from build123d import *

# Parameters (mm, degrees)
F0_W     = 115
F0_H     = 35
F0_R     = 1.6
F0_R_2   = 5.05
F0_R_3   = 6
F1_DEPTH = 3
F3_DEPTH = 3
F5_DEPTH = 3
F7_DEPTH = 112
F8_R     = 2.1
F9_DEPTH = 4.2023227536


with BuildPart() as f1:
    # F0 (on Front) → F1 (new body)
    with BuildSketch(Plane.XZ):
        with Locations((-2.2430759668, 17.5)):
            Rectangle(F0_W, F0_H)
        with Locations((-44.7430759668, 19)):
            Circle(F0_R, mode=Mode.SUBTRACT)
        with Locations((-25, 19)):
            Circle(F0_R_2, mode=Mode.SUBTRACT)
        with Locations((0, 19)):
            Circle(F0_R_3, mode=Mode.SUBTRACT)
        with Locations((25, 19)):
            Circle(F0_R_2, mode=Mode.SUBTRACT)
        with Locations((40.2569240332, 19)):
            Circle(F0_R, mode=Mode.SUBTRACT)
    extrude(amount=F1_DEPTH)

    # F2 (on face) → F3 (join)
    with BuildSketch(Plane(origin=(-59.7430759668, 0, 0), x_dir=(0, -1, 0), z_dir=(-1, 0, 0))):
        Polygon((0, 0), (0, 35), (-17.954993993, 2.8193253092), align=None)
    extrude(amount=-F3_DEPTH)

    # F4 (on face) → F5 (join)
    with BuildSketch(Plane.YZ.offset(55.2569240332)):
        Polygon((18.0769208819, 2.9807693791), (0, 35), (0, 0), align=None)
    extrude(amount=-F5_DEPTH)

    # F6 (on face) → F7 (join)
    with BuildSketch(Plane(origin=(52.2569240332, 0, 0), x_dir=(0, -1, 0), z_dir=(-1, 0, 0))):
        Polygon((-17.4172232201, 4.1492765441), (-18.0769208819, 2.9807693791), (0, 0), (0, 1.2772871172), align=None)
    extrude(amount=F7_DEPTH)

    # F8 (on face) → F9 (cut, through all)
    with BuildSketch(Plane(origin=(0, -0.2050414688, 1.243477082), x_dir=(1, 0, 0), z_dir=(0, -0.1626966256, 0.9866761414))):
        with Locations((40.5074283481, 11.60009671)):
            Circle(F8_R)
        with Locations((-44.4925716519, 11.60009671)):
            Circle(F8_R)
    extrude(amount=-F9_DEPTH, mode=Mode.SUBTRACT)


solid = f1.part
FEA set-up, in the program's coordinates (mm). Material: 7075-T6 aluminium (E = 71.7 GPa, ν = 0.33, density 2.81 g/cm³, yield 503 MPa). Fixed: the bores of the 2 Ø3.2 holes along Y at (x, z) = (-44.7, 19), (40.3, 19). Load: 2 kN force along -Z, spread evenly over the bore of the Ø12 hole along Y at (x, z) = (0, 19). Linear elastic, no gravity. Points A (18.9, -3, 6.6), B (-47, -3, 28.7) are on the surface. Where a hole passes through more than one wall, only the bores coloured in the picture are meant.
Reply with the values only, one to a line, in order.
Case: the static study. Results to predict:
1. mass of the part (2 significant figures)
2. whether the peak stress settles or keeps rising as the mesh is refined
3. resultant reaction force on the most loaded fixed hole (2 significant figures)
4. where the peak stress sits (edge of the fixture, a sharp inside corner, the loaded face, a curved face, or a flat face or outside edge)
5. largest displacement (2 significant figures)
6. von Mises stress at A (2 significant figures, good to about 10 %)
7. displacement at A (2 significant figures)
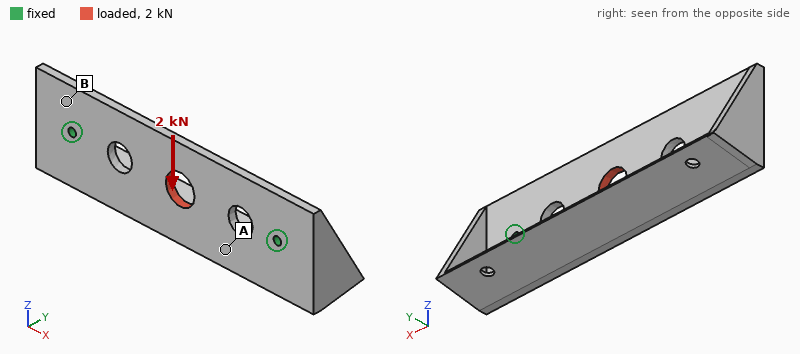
44 g
keeps rising
1.1 kN
edge of the fixture
67 µm
30 MPa
36 µm
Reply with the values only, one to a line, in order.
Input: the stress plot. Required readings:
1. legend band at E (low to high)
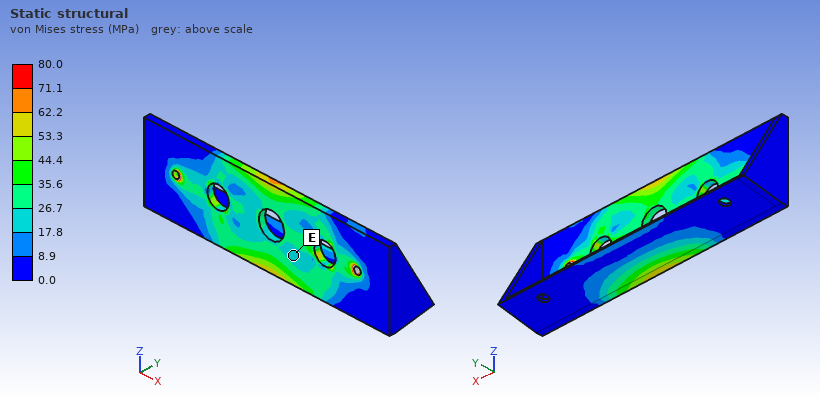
17.8 to 26.7 MPa
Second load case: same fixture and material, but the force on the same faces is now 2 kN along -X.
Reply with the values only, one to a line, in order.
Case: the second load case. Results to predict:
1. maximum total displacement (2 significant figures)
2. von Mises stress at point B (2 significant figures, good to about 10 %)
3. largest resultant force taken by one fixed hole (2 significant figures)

11 µm
6.9 MPa
1.0 kN
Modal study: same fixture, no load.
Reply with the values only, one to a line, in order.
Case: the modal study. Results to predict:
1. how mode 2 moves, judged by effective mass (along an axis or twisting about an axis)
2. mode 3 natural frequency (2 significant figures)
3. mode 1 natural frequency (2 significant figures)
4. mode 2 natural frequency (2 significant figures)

along Y
3100 Hz
2200 Hz
2500 Hz
